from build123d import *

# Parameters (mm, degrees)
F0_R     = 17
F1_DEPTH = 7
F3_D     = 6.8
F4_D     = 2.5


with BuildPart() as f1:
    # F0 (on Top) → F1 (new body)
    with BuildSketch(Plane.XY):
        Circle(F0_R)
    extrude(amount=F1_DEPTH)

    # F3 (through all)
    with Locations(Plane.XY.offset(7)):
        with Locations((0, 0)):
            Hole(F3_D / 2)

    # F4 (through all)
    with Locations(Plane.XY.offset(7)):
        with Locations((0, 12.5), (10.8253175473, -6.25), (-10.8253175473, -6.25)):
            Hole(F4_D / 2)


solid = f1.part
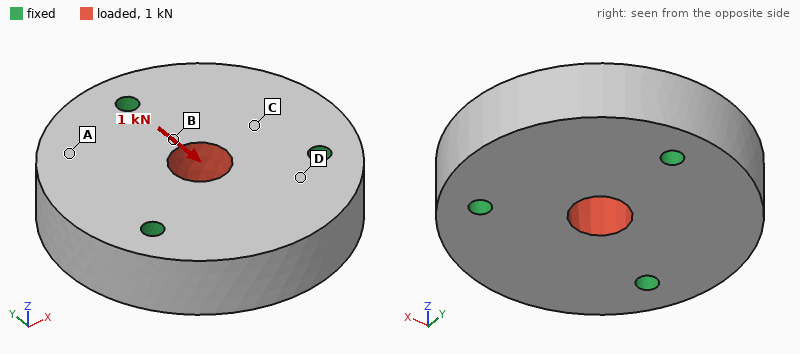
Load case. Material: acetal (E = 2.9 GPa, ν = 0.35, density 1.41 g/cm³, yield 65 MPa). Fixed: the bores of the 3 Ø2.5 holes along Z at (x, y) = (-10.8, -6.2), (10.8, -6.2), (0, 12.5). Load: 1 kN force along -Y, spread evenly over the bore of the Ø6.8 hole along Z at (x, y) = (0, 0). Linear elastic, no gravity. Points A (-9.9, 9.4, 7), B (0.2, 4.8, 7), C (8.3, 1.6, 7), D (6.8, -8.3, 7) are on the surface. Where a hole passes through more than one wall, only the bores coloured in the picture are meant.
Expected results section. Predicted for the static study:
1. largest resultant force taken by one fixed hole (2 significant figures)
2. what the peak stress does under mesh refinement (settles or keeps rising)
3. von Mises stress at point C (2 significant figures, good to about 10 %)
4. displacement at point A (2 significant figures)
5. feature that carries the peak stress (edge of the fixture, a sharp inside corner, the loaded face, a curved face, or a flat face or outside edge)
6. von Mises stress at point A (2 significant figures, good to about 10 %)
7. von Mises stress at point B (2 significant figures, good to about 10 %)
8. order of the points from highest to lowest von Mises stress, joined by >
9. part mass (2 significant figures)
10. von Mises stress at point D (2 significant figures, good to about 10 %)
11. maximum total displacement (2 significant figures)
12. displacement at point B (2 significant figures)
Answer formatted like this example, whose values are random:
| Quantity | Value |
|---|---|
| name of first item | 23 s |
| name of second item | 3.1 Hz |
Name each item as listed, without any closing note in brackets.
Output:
| Quantity | Value |
|---|---|
| largest resultant force taken by one fixed hole | 350 N |
| what the peak stress does under mesh refinement | keeps rising |
| von Mises stress at point C | 2.5 MPa |
| displacement at point A | 12 µm |
| feature that carries the peak stress | edge of the fixture |
| von Mises stress at point A | 1.3 MPa |
| von Mises stress at point B | 8.0 MPa |
| order of the points from highest to lowest von Mises stress, joined by > | B > D > C > A |
| part mass | 8.5 g |
| von Mises stress at point D | 4.4 MPa |
| maximum total displacement | 34 µm |
| displacement at point B | 18 µm |
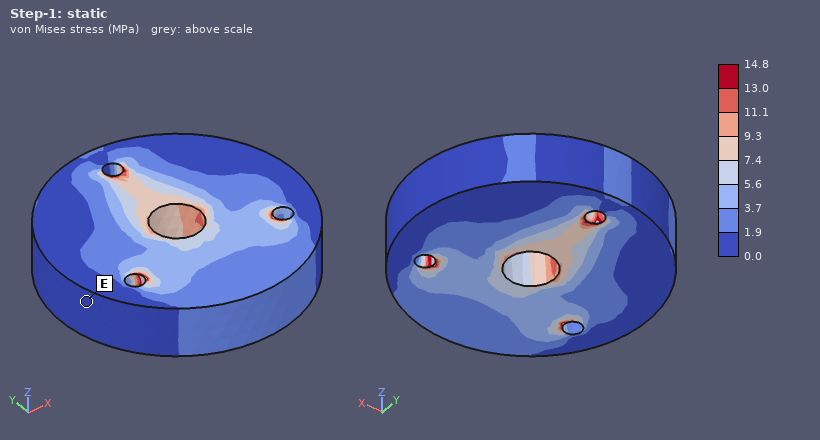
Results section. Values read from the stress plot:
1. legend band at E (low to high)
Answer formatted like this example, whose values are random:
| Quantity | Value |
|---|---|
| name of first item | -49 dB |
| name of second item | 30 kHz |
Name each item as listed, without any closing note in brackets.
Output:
| Quantity | Value |
|---|---|
| legend band at E | 0.0 to 1.9 MPa |
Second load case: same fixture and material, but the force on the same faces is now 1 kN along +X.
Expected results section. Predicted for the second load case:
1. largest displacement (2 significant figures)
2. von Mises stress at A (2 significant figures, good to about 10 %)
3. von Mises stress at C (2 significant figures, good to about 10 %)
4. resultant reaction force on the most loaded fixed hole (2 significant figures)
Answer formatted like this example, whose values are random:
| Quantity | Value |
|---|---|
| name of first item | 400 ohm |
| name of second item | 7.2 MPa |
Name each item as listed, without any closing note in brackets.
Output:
| Quantity | Value |
|---|---|
| largest displacement | 32 µm |
| von Mises stress at A | 2.6 MPa |
| von Mises stress at C | 3.9 MPa |
| resultant reaction force on the most loaded fixed hole | 340 N |
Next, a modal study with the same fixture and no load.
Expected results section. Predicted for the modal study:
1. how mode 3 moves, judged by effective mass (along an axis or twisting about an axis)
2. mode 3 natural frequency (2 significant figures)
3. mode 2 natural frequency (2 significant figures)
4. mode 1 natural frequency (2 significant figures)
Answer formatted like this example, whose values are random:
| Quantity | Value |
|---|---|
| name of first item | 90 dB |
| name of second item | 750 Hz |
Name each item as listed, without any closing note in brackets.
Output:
| Quantity | Value |
|---|---|
| how mode 3 moves, judged by effective mass | along Z |
| mode 3 natural frequency | 10 kHz |
| mode 2 natural frequency | 8900 Hz |
| mode 1 natural frequency | 8900 Hz |
